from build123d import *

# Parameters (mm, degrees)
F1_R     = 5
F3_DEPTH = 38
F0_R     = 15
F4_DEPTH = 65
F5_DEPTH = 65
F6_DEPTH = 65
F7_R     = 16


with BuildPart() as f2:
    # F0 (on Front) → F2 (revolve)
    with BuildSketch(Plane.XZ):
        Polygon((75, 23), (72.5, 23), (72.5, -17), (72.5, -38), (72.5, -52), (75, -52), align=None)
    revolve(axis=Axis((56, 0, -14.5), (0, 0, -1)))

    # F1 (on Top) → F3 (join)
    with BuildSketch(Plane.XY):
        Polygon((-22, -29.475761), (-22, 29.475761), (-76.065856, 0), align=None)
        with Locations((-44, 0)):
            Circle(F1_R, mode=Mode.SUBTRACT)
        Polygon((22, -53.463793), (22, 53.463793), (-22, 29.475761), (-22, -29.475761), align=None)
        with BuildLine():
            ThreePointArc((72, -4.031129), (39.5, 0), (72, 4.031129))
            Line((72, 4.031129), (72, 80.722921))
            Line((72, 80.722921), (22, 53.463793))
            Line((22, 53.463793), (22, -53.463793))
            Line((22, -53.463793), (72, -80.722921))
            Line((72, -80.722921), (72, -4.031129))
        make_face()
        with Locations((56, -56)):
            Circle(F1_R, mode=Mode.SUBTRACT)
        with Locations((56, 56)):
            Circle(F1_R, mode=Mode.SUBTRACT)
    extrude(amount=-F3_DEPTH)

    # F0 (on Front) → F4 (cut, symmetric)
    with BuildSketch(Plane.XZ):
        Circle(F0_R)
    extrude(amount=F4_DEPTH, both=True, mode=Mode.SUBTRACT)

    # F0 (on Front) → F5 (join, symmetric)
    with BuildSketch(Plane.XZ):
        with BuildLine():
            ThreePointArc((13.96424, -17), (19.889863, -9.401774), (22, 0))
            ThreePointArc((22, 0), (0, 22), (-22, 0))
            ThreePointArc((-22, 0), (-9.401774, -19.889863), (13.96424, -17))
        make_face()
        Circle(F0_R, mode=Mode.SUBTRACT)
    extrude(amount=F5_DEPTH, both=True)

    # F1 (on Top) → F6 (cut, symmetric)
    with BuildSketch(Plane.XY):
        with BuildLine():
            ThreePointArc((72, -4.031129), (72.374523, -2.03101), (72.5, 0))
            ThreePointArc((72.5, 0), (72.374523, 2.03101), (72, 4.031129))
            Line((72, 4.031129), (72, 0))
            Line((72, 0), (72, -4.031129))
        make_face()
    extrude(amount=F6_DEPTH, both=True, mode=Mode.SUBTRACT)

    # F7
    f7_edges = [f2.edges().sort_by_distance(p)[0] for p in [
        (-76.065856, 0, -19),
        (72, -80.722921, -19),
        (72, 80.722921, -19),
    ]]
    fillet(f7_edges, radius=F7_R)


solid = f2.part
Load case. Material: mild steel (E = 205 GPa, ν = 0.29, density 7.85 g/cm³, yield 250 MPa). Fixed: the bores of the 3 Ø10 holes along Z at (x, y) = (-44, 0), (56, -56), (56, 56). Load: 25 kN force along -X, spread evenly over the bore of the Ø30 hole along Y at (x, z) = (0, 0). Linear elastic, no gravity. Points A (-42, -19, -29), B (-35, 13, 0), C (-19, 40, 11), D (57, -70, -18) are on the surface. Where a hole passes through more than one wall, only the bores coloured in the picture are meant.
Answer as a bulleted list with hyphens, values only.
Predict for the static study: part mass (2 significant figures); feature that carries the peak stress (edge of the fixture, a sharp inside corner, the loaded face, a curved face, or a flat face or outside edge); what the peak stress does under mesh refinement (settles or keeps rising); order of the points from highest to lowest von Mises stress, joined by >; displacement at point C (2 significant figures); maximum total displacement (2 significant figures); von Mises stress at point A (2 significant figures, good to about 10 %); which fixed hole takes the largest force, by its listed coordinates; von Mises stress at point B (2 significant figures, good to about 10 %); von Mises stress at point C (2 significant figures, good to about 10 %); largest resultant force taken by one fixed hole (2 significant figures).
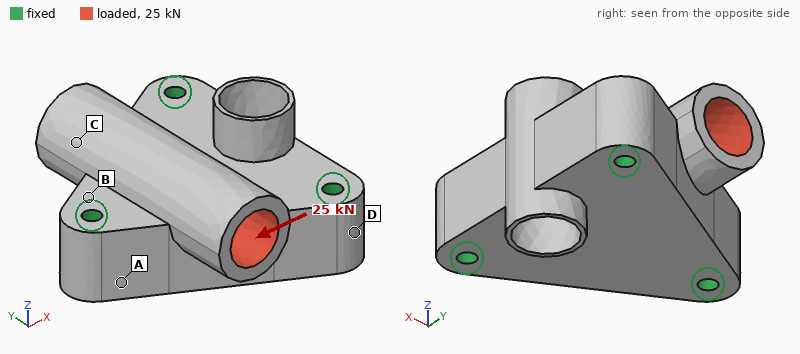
- 3.5 kg
- a sharp inside corner
- keeps rising
- C > B > A > D
- 8.6 µm
- 11 µm
- 5.5 MPa
- (-44, 0)
- 11 MPa
- 14 MPa
- 13 kN
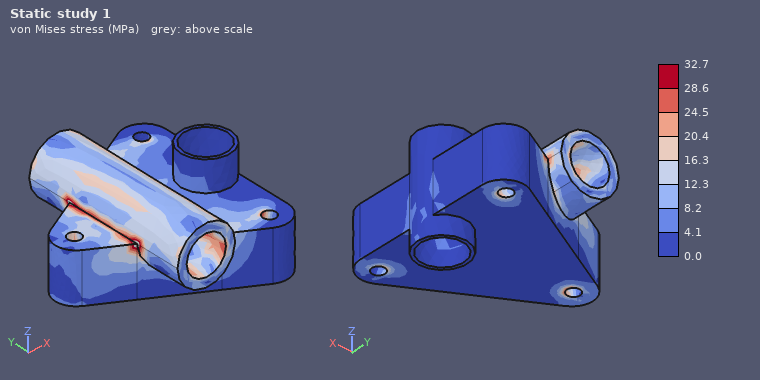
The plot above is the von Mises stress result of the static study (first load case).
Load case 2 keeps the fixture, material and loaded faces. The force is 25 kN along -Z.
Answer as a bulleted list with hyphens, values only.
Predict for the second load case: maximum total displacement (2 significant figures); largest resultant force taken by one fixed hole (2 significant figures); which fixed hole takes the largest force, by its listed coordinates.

- 11 µm
- 13 kN
- (-44, 0)
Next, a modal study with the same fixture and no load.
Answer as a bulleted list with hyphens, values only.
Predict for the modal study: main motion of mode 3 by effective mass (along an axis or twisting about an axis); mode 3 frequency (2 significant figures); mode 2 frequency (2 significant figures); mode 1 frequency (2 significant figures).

- along X
- 9200 Hz
- 7400 Hz
- 7300 Hz
